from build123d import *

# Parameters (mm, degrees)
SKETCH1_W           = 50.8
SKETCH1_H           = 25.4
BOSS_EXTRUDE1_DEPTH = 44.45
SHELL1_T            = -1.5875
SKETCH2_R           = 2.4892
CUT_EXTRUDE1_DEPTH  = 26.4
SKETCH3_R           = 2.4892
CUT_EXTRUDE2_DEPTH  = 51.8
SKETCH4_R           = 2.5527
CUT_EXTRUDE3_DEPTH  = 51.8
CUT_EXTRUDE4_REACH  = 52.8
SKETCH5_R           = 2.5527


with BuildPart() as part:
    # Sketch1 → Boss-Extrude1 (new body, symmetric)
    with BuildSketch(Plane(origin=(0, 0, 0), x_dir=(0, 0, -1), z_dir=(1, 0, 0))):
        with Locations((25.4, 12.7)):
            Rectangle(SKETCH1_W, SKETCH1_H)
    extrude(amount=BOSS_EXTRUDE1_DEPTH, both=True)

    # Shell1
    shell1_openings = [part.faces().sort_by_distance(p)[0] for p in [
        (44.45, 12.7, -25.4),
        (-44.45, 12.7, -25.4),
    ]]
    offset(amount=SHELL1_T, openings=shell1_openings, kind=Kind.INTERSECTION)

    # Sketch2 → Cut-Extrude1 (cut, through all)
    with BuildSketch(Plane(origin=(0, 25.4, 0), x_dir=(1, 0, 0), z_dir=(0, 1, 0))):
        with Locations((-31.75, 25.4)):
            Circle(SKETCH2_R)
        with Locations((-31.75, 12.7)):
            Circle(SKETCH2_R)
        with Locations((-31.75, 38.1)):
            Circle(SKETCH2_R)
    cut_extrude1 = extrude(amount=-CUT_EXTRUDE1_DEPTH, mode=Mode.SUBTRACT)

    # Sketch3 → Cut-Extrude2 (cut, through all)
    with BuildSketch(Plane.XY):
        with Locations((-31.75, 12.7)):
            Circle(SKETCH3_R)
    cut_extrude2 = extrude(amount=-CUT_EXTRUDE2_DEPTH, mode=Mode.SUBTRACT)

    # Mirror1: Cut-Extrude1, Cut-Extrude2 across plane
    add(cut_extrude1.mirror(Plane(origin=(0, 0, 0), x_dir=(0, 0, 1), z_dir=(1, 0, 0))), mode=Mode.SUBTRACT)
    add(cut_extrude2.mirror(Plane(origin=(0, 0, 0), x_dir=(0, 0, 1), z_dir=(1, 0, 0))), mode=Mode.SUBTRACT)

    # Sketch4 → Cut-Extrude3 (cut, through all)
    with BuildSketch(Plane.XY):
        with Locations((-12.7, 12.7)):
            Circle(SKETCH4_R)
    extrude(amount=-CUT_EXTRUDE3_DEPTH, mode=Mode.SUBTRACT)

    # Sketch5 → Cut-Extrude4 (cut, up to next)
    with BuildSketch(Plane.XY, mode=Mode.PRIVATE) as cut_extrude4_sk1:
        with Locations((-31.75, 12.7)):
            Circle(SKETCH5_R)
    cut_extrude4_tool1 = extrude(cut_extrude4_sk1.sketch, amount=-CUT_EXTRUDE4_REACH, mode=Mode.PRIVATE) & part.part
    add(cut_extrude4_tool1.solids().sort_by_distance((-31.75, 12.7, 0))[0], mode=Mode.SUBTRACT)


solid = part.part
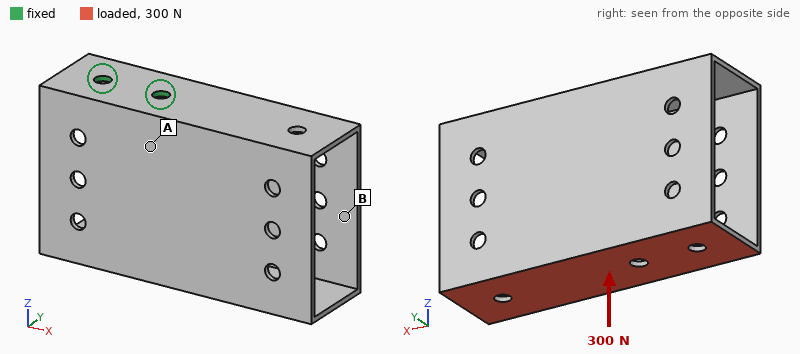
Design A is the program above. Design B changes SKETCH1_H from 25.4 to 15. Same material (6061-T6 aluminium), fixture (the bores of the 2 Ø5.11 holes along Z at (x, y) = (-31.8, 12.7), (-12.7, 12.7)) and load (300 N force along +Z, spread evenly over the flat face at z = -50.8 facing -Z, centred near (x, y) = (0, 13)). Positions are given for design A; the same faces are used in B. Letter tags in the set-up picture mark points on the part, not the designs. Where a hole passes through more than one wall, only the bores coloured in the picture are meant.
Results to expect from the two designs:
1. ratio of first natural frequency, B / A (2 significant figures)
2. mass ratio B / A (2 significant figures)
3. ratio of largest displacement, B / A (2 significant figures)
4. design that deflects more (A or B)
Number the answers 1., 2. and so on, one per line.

1. 1.4
2. 0.85
3. 0.29
4. A
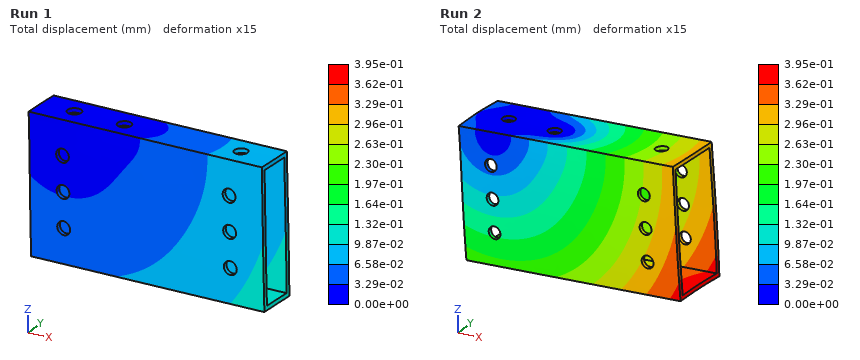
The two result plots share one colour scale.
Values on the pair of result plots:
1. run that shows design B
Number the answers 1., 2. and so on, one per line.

1. Run 1
